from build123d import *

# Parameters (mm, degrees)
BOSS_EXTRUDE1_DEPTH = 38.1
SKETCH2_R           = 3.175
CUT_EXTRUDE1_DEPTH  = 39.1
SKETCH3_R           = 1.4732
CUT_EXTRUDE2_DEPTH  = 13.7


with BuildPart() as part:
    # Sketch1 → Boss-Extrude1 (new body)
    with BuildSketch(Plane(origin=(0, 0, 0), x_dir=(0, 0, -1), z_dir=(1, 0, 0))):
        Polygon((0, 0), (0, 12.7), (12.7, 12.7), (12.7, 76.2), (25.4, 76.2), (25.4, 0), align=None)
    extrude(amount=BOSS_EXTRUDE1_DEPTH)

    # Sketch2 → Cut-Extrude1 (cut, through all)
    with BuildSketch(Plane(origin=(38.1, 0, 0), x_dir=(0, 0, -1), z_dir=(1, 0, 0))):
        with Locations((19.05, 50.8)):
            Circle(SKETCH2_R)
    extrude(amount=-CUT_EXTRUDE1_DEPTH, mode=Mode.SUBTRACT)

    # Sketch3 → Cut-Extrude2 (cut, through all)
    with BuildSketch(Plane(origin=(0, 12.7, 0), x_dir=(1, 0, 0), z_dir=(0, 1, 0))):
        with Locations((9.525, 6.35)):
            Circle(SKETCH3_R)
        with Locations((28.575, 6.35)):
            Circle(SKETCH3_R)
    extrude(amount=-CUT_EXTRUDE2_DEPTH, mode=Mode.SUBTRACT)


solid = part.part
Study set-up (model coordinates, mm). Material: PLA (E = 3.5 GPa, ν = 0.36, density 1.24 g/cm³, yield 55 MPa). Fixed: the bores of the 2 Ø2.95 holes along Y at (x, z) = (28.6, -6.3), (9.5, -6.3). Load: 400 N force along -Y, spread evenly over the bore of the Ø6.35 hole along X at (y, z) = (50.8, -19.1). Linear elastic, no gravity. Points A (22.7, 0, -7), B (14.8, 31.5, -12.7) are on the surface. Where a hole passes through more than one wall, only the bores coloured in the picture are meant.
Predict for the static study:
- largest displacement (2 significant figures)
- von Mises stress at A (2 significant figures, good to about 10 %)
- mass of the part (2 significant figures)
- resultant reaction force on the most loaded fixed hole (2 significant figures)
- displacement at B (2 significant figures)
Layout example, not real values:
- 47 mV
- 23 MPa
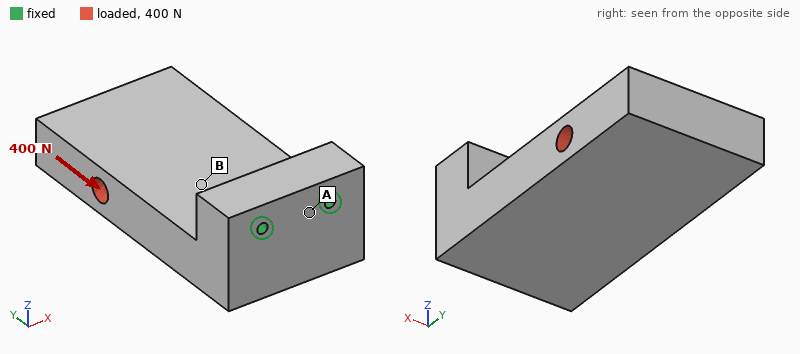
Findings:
- 0.18 mm
- 2.0 MPa
- 52 g
- 200 N
- 0.064 mm
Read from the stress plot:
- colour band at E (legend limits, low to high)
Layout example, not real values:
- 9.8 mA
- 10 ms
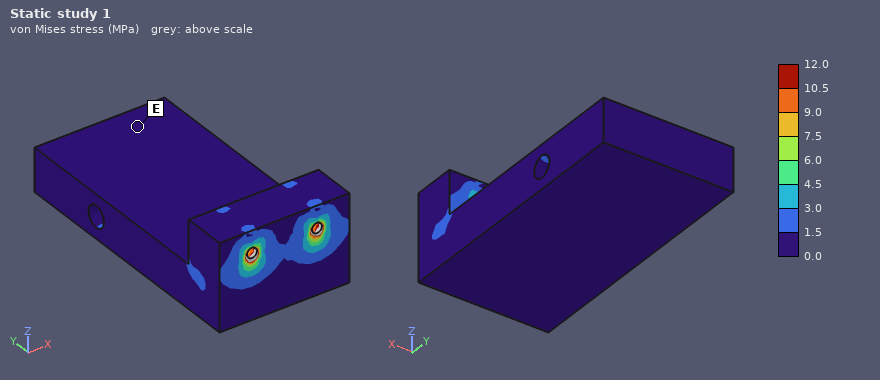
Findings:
- 0.0 to 1.5 MPa
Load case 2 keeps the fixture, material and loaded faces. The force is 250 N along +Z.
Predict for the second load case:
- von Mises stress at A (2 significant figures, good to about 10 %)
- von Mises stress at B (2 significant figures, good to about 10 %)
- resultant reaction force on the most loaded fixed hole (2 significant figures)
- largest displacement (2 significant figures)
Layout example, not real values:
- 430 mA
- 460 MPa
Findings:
- 5.0 MPa
- 4.6 MPa
- 140 N
- 1.0 mm
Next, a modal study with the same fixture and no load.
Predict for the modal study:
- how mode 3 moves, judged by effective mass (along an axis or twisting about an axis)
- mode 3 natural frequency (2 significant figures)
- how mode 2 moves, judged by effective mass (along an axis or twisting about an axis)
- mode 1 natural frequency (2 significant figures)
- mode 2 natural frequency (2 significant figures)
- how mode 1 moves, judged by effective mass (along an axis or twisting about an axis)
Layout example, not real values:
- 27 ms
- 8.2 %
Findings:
- twisting about Y
- 2200 Hz
- along X
- 550 Hz
- 1000 Hz
- along Z
